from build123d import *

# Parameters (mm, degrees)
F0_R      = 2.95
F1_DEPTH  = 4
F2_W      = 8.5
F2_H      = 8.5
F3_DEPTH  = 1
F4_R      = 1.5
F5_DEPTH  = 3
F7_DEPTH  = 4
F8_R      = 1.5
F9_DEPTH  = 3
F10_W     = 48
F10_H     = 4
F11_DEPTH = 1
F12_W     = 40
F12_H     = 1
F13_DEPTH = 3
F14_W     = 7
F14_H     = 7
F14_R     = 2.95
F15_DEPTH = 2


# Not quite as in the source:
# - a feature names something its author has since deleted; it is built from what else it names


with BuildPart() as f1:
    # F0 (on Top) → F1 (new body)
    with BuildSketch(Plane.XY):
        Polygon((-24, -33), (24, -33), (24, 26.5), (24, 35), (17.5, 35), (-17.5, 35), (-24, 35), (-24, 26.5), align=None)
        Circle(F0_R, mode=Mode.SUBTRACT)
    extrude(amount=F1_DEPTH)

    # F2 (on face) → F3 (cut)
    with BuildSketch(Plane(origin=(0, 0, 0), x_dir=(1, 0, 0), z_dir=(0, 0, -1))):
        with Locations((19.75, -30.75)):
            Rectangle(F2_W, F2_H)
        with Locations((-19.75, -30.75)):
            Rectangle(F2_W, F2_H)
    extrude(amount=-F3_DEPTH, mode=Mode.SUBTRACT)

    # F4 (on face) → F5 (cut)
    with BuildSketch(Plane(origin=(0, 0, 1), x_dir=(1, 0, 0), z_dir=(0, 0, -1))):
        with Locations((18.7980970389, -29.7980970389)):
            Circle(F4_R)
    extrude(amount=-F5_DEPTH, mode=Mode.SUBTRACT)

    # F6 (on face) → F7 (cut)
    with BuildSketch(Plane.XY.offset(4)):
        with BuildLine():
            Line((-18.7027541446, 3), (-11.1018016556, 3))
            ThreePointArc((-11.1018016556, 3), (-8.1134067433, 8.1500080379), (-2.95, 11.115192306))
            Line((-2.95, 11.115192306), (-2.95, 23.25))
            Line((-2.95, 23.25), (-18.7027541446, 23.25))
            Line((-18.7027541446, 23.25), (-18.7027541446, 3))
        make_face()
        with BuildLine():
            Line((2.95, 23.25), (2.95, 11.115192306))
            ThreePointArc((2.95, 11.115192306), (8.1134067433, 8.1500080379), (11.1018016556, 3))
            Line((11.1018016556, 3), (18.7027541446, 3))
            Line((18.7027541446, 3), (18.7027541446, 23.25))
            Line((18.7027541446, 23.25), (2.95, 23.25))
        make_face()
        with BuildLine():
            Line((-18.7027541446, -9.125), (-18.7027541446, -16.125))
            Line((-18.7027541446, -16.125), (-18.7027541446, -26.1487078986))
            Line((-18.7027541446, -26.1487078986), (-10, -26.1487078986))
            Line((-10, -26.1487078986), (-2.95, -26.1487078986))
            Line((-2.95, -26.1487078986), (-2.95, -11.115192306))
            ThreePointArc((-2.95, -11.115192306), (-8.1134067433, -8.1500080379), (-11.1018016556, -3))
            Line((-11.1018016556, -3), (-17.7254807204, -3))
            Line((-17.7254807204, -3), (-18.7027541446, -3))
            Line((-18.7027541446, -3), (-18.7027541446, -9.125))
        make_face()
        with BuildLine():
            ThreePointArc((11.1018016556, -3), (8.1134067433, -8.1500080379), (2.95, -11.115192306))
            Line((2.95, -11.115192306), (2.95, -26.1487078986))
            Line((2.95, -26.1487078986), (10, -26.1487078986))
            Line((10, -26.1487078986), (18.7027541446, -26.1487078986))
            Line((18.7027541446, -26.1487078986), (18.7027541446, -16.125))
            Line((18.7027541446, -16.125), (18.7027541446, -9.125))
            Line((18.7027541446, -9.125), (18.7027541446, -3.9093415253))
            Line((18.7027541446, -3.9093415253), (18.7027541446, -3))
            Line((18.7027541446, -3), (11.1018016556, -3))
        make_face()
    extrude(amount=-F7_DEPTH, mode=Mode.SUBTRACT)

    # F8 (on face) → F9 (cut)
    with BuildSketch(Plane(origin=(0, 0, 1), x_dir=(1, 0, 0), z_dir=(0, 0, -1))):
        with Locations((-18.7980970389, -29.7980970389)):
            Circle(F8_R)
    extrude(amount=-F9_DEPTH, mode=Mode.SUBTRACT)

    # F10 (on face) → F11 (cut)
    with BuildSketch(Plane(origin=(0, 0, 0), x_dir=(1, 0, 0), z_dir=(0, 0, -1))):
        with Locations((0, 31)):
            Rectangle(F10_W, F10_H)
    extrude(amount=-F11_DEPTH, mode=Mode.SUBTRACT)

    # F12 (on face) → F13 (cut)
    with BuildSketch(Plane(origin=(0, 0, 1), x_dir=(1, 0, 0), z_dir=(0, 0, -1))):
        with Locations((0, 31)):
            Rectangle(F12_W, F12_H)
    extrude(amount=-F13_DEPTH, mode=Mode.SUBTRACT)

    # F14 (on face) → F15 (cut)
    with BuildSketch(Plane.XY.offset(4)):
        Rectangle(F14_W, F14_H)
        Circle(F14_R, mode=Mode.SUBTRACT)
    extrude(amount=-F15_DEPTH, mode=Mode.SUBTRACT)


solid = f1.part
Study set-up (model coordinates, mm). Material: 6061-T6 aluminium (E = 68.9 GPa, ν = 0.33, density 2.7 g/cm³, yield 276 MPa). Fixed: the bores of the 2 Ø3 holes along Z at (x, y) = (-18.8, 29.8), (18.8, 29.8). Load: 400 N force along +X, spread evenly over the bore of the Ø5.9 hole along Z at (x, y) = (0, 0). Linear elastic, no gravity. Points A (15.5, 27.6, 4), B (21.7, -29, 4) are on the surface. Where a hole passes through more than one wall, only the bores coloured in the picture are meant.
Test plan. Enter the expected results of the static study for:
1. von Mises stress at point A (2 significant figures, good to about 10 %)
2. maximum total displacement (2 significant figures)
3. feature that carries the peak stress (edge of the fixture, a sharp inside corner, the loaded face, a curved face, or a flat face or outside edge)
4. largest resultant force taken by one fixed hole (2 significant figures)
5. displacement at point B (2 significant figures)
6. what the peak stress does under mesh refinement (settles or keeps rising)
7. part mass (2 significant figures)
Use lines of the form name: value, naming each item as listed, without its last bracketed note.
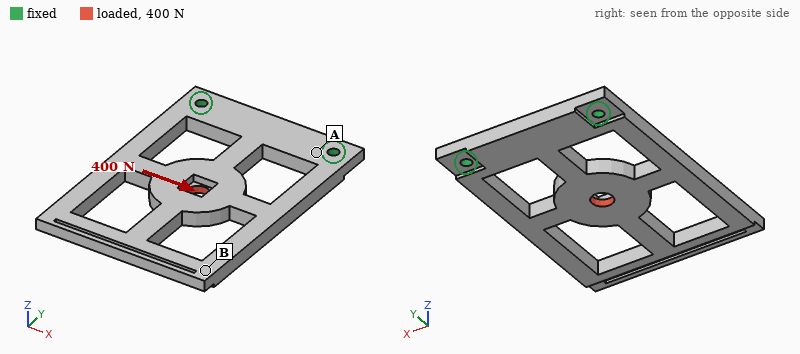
von Mises stress at point A: 14 MPa
maximum total displacement: 50 µm
feature that carries the peak stress: a sharp inside corner
largest resultant force taken by one fixed hole: 360 N
displacement at point B: 47 µm
what the peak stress does under mesh refinement: keeps rising
part mass: 21 g
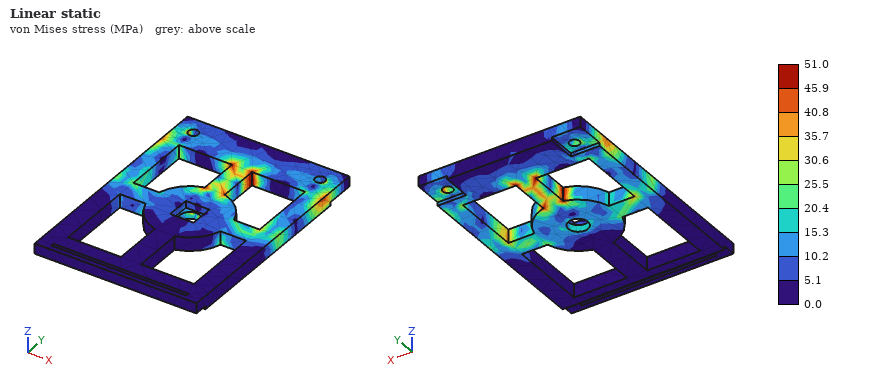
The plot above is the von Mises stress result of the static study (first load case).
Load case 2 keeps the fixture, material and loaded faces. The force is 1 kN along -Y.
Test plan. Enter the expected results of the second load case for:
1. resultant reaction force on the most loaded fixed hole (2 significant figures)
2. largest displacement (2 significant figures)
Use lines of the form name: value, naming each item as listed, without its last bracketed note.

resultant reaction force on the most loaded fixed hole: 510 N
largest displacement: 0.24 mm
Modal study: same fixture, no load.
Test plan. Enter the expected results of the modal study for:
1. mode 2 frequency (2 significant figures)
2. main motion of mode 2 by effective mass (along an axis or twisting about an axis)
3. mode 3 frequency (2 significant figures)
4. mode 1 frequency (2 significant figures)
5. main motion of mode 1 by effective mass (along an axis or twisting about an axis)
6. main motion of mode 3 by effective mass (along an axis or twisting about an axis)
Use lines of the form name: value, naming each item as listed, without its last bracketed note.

mode 2 frequency: 1800 Hz
main motion of mode 2 by effective mass: twisting about Y
mode 3 frequency: 3700 Hz
mode 1 frequency: 650 Hz
main motion of mode 1 by effective mass: along Z
main motion of mode 3 by effective mass: along X
